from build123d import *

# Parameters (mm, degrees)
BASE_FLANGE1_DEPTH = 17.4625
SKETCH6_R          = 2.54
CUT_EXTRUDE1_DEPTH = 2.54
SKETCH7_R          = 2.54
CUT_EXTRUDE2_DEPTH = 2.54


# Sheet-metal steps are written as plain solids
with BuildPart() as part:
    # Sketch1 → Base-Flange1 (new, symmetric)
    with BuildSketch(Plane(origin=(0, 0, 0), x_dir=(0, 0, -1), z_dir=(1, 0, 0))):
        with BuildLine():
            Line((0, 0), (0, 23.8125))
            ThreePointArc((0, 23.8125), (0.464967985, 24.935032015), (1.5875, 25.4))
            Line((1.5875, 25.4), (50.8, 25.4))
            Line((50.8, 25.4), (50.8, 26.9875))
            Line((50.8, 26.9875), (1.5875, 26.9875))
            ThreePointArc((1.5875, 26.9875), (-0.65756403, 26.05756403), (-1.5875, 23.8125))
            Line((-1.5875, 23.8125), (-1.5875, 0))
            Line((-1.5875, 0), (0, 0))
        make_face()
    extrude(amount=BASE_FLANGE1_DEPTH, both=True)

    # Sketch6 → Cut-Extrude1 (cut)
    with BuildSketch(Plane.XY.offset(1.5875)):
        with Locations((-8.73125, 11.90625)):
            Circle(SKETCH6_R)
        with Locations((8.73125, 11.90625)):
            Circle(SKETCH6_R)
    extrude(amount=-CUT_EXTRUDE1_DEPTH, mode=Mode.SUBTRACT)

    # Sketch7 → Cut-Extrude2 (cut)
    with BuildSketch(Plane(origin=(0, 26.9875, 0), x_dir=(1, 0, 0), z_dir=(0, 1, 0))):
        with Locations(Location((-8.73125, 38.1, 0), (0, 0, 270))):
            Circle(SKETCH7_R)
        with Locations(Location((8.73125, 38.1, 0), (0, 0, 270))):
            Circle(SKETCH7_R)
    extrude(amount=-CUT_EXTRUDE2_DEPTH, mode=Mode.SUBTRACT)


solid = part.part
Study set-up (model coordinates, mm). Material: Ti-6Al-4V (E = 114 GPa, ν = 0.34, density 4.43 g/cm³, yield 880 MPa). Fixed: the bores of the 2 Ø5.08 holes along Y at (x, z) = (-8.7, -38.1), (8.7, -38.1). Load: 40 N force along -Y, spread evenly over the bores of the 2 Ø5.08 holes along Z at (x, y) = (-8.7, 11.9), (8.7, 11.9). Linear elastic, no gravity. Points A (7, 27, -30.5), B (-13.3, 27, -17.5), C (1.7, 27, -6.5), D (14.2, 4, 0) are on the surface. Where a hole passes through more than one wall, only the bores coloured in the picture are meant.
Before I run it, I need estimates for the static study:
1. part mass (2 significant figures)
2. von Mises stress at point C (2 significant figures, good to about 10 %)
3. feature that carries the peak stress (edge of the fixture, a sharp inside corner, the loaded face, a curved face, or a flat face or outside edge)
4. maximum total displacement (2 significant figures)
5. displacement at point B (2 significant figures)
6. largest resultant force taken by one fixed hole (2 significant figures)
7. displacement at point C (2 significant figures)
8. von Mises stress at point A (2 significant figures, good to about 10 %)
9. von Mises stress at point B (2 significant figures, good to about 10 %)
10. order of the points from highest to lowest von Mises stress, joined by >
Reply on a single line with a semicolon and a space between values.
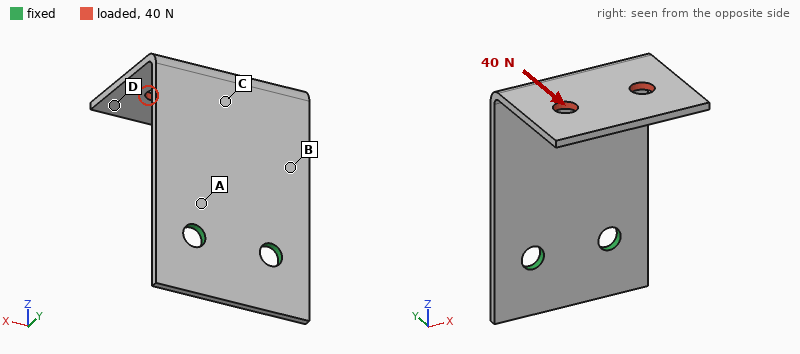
18 g; 18 MPa; a flat face or outside edge; 0.73 mm; 0.16 mm; 20 N; 0.35 mm; 77 MPa; 49 MPa; A > B > C > D
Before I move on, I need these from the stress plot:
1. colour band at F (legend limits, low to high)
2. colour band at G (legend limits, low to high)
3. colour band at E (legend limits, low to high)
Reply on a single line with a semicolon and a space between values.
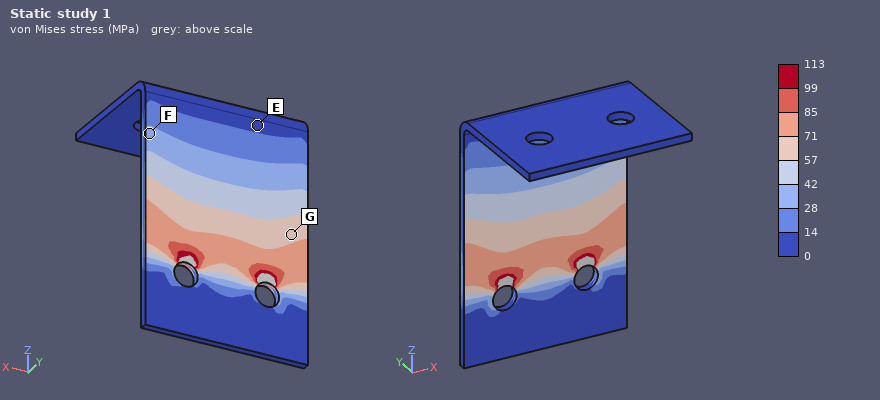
28 to 42 MPa; 57 to 71 MPa; 0 to 14 MPa
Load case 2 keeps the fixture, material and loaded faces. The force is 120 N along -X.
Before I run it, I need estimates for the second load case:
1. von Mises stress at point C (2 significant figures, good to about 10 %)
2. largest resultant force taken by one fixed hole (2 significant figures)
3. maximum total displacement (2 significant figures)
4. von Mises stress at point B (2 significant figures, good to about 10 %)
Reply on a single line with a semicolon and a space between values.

73 MPa; 240 N; 0.72 mm; 82 MPa
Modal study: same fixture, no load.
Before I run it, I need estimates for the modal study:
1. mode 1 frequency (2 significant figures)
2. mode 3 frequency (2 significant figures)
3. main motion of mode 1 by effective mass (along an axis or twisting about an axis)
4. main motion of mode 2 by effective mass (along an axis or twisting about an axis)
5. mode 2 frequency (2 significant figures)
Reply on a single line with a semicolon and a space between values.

440 Hz; 1400 Hz; along Y; along X; 900 Hz
